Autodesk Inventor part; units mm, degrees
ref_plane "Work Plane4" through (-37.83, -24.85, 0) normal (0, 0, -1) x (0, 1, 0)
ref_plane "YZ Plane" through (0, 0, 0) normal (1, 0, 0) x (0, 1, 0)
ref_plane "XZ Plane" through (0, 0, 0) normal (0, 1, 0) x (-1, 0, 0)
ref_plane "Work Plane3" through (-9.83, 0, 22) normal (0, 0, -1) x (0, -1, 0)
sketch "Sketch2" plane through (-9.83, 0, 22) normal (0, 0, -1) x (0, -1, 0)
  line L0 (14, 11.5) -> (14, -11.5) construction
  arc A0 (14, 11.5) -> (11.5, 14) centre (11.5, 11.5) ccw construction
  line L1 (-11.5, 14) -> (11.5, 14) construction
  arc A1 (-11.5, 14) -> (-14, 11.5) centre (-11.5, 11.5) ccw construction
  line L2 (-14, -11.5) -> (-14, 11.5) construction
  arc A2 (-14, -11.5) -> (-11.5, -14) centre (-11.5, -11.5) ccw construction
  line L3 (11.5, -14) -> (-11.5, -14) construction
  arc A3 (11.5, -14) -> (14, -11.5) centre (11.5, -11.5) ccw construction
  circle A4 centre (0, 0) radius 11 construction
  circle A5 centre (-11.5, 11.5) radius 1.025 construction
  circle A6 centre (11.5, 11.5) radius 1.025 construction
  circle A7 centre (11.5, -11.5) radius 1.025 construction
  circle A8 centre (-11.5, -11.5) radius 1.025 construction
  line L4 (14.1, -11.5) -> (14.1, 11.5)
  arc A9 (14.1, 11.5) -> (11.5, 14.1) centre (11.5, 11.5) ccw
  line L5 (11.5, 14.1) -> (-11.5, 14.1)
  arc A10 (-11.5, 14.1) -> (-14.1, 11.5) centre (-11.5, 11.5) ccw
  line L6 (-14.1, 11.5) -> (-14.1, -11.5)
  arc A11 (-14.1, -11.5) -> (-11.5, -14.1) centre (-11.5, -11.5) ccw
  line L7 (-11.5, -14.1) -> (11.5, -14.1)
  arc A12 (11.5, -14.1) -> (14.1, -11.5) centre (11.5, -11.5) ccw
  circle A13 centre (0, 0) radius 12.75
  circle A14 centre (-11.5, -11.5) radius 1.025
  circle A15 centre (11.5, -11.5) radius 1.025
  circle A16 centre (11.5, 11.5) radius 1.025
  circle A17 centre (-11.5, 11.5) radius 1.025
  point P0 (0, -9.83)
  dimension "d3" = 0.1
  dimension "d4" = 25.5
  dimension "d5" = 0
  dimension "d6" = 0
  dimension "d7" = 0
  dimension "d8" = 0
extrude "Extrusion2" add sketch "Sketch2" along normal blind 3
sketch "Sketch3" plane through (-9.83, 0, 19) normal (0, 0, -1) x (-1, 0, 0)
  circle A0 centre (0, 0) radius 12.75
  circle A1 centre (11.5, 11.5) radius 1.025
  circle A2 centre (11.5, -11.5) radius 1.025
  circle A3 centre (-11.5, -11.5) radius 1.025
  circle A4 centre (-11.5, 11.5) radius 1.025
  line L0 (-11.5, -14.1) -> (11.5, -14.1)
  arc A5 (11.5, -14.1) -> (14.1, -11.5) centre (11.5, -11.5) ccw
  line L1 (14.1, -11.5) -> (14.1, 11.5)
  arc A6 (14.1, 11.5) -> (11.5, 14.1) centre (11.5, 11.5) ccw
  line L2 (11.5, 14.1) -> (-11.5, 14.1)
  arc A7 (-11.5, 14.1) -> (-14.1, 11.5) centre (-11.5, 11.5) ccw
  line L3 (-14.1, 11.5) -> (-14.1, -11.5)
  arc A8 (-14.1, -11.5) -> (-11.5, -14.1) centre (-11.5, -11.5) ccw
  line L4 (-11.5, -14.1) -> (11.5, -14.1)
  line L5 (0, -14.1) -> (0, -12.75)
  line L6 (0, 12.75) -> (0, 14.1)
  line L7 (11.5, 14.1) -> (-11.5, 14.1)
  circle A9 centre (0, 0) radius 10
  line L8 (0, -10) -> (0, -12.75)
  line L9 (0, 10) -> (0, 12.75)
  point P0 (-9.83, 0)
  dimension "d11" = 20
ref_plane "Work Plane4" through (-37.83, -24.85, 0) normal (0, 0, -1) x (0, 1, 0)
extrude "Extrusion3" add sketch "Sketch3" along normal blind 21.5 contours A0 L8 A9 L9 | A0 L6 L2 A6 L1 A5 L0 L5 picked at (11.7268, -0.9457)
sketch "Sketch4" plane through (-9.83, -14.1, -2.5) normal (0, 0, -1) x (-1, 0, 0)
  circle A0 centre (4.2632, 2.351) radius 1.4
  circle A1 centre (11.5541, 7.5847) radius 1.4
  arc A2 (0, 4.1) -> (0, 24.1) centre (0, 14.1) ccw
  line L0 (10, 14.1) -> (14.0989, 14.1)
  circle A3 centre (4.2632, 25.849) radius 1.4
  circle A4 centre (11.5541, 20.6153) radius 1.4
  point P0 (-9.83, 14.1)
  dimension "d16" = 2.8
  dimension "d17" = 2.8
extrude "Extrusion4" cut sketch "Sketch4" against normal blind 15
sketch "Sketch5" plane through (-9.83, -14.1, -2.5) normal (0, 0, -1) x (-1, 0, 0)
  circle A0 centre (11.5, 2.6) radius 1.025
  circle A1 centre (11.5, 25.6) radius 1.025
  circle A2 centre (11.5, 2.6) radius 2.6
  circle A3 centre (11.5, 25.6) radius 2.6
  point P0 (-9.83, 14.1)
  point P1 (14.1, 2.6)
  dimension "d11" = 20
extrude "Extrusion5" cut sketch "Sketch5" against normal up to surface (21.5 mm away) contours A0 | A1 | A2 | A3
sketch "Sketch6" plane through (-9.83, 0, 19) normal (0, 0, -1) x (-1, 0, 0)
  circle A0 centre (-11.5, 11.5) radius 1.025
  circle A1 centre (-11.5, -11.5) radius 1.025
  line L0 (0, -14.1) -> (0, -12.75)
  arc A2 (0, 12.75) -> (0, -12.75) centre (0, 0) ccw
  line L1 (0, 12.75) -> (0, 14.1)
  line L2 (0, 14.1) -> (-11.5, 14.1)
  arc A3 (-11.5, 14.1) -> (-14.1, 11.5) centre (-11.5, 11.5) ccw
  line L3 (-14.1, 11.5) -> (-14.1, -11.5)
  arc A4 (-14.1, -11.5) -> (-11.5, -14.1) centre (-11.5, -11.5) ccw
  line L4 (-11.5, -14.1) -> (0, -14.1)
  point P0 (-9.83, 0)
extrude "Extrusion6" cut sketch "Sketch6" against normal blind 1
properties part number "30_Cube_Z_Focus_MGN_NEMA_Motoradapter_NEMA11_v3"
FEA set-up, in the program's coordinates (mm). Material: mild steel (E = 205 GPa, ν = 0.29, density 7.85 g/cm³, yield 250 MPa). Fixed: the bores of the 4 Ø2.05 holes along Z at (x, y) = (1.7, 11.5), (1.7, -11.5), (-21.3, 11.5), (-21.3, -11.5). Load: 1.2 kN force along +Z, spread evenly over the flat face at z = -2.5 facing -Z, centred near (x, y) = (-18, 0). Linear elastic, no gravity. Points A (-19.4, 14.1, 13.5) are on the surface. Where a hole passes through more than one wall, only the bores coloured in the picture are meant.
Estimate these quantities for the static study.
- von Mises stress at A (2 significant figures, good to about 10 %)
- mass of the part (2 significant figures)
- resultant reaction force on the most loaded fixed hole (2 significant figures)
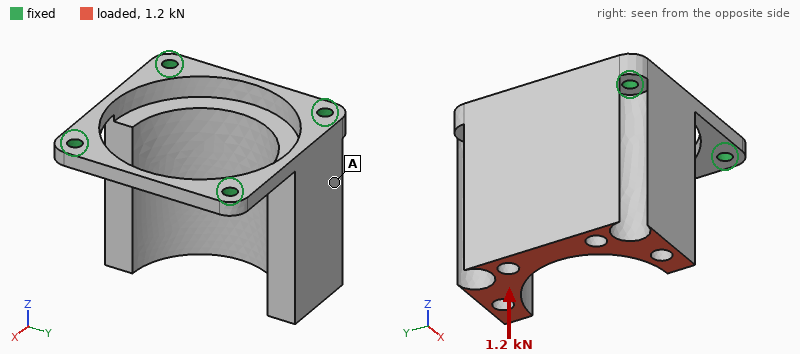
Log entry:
21 MPa
35 g
590 N
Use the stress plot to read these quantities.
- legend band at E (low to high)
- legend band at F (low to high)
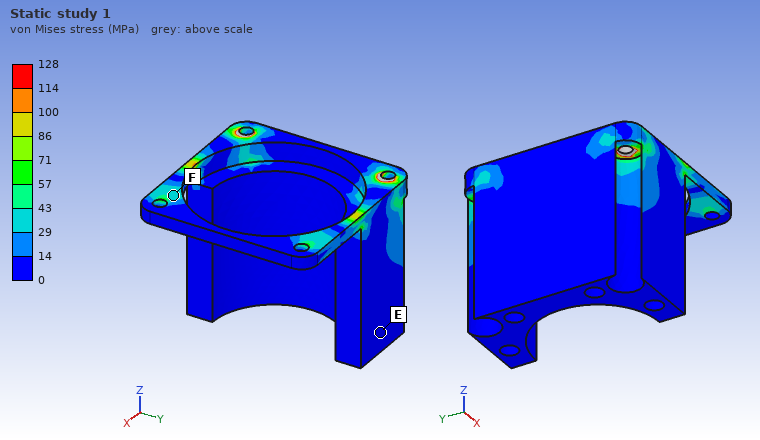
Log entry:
0 to 14 MPa
29 to 43 MPa
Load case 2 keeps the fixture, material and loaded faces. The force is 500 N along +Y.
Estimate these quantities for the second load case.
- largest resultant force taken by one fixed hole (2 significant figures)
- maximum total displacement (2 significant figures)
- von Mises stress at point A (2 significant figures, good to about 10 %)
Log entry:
570 N
10 µm
24 MPa
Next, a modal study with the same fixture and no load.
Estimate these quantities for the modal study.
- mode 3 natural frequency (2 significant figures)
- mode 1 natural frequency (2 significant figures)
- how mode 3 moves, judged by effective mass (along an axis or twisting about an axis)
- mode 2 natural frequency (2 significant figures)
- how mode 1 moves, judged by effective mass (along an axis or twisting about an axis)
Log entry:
14 kHz
4100 Hz
along Y
8800 Hz
along X
